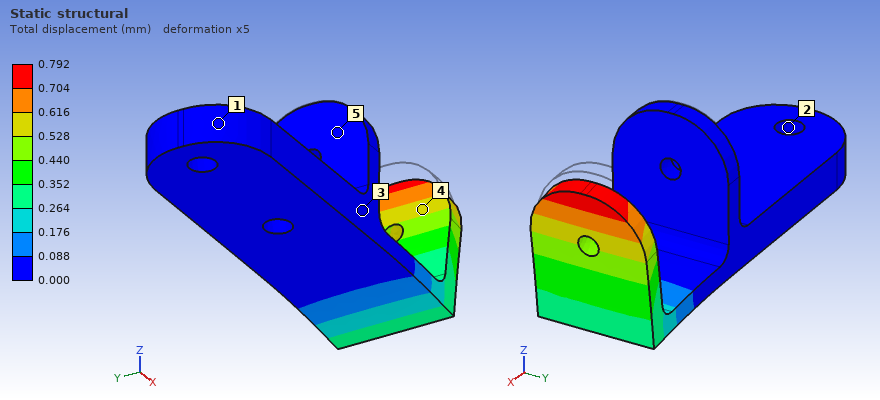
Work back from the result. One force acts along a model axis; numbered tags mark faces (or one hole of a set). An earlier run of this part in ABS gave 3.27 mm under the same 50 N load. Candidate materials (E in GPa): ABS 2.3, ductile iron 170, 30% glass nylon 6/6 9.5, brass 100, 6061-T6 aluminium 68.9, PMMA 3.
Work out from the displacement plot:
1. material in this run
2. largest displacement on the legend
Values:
30% glass nylon 6/6
0.792 mm
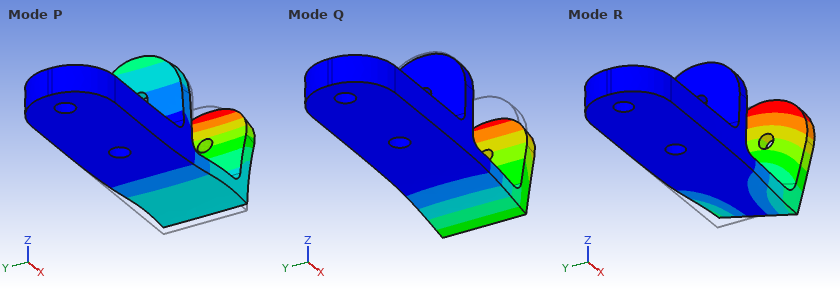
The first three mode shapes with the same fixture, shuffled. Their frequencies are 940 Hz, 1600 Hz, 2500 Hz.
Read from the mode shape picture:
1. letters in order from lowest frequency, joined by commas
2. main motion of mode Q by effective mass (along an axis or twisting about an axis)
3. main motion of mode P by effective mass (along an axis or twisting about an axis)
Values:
Q, R, P
along Z
along Z
